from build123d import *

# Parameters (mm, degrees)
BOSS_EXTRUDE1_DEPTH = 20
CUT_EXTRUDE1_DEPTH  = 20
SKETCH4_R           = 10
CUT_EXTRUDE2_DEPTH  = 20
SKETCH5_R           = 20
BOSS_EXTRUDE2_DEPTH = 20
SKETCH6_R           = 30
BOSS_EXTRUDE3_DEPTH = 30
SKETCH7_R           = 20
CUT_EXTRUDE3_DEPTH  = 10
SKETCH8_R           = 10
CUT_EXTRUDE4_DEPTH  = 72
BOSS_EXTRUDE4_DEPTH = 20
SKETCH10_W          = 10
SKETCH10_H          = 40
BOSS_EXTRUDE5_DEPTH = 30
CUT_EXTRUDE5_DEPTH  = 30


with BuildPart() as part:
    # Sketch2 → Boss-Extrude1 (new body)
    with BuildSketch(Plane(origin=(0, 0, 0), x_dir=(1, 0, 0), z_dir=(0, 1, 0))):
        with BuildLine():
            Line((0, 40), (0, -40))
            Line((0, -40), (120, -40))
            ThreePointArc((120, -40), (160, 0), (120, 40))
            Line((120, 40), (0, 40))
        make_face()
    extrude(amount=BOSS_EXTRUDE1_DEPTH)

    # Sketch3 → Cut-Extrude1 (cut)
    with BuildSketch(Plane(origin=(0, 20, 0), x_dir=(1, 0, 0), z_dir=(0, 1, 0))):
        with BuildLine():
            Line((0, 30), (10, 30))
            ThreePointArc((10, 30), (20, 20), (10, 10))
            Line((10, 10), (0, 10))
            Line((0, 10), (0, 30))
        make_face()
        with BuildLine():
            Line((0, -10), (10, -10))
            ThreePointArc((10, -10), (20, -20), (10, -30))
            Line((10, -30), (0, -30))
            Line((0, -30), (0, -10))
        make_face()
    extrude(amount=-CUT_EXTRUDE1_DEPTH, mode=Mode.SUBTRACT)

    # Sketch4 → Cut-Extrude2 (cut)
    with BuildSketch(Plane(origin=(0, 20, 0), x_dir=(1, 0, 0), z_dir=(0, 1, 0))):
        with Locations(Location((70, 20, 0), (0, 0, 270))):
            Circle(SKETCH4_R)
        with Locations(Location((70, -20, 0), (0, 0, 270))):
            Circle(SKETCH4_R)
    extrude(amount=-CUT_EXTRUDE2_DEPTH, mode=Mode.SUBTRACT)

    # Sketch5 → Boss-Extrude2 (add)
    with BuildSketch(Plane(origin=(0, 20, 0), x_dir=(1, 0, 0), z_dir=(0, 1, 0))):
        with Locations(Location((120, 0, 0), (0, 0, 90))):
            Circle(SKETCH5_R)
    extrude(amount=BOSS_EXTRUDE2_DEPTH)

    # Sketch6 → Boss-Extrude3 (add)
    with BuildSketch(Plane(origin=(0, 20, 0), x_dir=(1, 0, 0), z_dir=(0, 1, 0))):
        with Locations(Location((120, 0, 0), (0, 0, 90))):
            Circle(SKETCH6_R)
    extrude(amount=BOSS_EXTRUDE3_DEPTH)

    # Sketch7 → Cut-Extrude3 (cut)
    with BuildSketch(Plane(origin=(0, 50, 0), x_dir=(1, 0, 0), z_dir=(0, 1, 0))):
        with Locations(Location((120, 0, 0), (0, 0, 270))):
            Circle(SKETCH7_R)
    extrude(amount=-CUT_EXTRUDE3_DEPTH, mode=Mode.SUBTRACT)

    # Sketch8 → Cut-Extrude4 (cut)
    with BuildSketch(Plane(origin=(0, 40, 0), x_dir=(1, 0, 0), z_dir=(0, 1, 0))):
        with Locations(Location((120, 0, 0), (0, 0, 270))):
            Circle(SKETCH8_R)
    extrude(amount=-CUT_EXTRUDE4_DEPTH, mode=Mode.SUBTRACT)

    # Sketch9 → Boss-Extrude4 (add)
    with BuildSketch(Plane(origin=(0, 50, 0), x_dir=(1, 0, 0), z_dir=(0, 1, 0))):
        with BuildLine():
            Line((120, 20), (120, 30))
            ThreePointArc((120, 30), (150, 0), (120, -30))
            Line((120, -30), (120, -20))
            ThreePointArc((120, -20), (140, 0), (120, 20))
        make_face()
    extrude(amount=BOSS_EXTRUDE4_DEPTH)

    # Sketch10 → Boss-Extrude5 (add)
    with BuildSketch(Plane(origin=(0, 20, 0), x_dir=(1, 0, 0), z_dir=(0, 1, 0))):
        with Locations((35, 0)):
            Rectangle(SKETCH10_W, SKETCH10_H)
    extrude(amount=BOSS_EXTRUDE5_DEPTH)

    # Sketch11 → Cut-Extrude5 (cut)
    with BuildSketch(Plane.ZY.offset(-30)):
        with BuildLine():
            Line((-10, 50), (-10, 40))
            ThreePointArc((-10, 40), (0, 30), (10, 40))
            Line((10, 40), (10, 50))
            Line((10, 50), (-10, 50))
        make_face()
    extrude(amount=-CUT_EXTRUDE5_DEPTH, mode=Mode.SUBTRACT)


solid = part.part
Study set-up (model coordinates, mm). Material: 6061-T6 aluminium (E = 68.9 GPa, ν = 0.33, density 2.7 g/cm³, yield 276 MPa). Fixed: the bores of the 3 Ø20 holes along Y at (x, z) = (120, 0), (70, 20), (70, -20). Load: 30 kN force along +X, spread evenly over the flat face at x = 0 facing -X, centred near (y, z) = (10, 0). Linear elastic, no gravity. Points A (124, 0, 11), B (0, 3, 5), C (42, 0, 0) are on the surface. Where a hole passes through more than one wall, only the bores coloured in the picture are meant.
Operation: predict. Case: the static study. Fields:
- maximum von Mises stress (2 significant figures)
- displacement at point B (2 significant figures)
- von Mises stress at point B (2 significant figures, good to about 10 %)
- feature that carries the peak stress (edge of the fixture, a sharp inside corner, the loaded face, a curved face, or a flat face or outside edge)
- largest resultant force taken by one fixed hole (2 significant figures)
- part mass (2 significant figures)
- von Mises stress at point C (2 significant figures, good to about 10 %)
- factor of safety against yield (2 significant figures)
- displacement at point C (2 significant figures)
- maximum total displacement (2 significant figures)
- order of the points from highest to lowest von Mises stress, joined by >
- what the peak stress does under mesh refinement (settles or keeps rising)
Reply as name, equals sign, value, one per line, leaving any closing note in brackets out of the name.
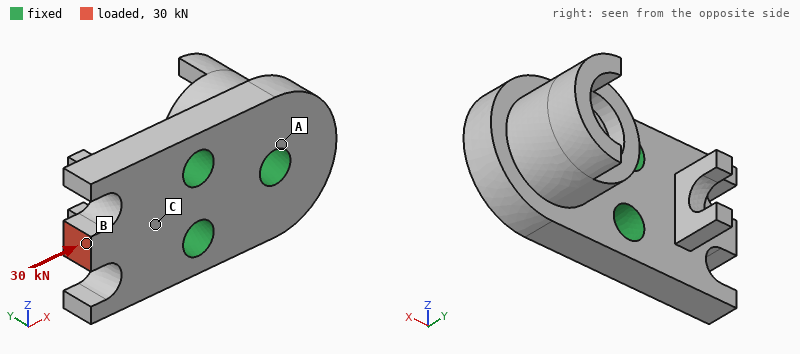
maximum von Mises stress = 110 MPa
displacement at point B = 42 µm
von Mises stress at point B = 75 MPa
feature that carries the peak stress = a curved face
largest resultant force taken by one fixed hole = 15 kN
part mass = 810 g
von Mises stress at point C = 35 MPa
factor of safety against yield = 2.4
displacement at point C = 10.0 µm
maximum total displacement = 43 µm
order of the points from highest to lowest von Mises stress, joined by > = B > C > A
what the peak stress does under mesh refinement = settles
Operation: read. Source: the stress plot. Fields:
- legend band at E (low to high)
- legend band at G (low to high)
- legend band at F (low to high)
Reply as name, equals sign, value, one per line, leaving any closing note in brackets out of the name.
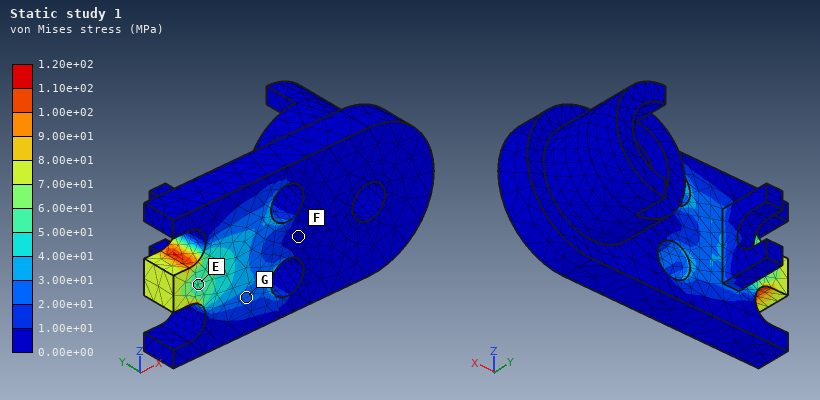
legend band at E = 5.00e+01 to 6.00e+01 MPa
legend band at G = 2.00e+01 to 3.00e+01 MPa
legend band at F = 0.00e+00 to 1.00e+01 MPa
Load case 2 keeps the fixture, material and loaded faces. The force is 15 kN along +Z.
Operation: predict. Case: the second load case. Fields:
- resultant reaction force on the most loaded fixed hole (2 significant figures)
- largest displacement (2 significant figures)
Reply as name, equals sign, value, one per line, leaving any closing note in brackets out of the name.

resultant reaction force on the most loaded fixed hole = 19 kN
largest displacement = 0.13 mm
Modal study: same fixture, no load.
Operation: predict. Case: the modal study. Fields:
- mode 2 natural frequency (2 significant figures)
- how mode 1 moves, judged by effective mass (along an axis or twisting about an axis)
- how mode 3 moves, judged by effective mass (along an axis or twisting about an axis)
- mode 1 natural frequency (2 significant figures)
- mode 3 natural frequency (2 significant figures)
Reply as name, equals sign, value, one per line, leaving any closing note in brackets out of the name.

mode 2 natural frequency = 6800 Hz
how mode 1 moves, judged by effective mass = along Y
how mode 3 moves, judged by effective mass = along Z
mode 1 natural frequency = 4400 Hz
mode 3 natural frequency = 9100 Hz
